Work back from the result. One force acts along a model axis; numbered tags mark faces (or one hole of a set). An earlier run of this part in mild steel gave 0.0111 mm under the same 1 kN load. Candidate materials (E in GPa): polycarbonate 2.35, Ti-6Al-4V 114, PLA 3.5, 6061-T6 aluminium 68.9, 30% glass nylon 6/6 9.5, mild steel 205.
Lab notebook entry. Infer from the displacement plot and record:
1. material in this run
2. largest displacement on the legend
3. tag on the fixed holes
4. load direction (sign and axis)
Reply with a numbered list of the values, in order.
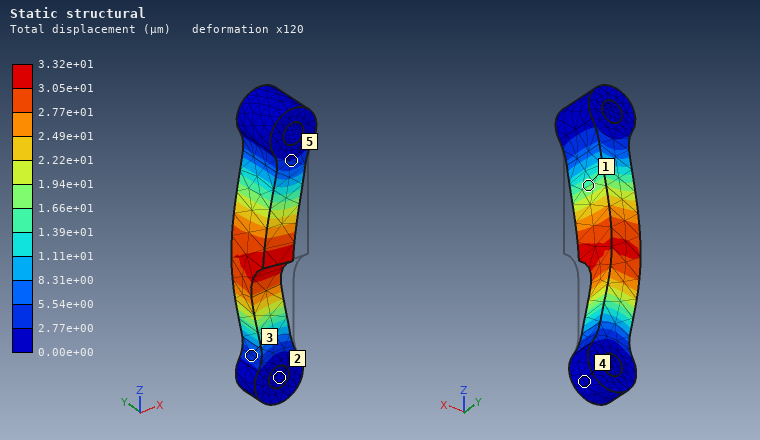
1. 6061-T6 aluminium
2. 3.32e+01 µm
3. 2
4. -X
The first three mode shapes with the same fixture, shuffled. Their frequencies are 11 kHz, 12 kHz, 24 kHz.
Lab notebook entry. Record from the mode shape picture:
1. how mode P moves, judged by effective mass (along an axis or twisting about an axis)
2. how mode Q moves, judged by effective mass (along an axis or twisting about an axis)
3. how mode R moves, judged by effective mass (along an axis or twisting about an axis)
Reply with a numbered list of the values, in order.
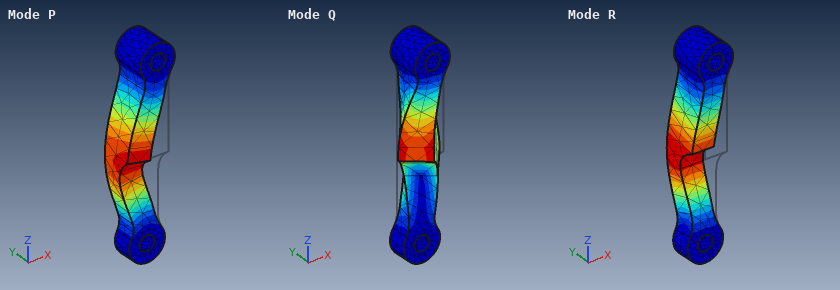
1. along X
2. twisting about Z
3. along Y
